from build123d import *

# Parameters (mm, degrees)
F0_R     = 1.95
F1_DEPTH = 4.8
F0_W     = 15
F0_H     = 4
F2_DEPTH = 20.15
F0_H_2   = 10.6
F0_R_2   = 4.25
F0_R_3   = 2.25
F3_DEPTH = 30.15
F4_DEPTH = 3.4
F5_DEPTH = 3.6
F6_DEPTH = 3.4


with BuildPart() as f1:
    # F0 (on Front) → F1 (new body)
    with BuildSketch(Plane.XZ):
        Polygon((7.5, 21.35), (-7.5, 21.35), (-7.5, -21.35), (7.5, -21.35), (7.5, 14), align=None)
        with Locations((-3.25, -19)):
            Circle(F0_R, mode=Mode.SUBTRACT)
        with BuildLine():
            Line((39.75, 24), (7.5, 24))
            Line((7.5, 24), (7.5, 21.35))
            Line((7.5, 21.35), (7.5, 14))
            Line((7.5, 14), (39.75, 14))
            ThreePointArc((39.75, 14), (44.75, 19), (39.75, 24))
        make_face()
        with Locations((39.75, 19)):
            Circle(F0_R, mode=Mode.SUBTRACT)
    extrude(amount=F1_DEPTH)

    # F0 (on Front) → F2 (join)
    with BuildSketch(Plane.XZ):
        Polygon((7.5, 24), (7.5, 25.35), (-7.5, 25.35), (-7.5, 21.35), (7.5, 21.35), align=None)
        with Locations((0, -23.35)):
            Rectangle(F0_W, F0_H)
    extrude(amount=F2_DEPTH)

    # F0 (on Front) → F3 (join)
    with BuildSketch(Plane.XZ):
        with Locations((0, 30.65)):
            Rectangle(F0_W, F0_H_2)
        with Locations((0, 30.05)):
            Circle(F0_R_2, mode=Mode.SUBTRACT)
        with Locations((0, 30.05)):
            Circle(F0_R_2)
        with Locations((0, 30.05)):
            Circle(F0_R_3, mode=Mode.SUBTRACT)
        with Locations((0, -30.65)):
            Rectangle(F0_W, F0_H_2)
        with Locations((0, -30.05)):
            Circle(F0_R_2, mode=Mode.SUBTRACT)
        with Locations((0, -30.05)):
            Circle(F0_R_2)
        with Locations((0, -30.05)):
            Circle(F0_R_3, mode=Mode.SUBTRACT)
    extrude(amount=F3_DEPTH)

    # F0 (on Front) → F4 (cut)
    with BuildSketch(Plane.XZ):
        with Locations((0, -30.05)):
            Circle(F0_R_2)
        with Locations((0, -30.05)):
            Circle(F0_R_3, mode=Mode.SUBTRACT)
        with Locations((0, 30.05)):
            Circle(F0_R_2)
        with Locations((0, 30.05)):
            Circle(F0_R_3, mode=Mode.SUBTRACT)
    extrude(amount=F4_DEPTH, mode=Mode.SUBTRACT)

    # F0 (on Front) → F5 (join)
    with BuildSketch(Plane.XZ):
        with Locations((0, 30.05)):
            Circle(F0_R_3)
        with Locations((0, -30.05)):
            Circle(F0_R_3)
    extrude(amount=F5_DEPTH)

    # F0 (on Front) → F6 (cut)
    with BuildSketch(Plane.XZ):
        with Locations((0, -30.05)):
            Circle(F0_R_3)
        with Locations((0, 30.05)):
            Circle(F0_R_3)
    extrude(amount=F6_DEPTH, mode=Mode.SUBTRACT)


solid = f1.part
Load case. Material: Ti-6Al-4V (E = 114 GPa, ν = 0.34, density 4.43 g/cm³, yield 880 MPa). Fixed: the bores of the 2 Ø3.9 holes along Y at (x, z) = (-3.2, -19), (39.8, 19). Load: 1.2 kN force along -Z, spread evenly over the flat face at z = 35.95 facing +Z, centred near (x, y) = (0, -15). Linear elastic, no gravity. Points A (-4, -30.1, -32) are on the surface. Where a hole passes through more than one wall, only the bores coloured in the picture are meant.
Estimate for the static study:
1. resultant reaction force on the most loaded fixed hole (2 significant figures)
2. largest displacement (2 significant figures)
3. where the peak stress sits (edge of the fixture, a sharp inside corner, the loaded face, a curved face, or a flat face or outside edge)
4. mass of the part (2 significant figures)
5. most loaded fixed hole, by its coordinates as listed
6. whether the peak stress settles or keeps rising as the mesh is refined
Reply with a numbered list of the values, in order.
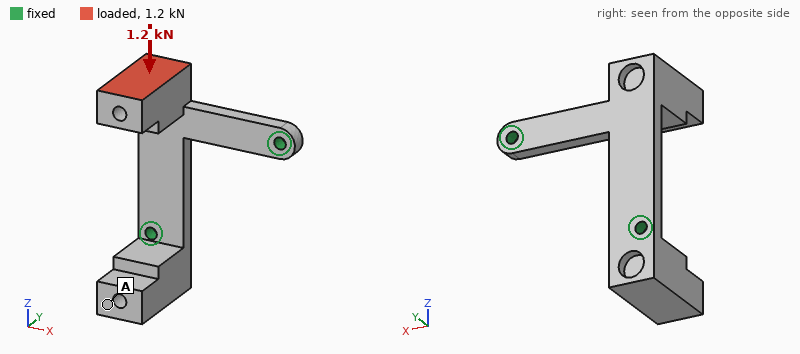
1. 1.2 kN
2. 0.79 mm
3. edge of the fixture
4. 69 g
5. (-3.2, -19)
6. keeps rising
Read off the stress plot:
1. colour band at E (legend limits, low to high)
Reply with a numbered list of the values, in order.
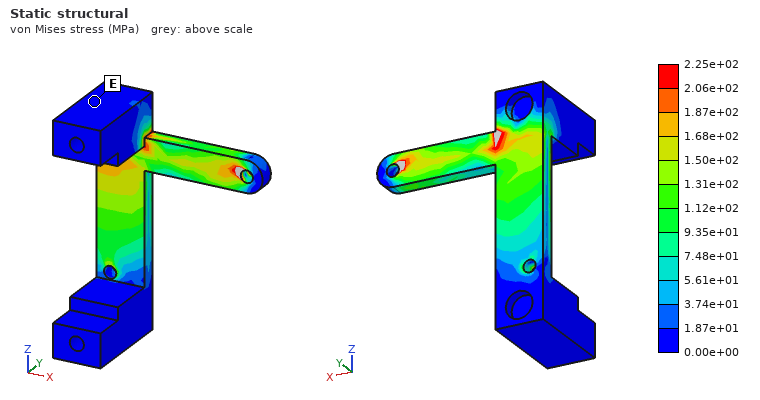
1. 0.00e+00 to 1.87e+01 MPa
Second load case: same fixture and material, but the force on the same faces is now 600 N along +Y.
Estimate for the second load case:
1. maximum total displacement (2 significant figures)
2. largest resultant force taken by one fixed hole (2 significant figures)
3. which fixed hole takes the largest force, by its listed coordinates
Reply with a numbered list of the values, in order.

1. 1.0 mm
2. 430 N
3. (39.8, 19)
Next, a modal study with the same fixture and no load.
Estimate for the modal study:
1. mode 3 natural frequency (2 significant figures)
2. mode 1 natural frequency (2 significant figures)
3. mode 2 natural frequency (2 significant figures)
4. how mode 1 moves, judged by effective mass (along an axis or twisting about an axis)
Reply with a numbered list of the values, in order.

1. 3300 Hz
2. 960 Hz
3. 2600 Hz
4. along Y
